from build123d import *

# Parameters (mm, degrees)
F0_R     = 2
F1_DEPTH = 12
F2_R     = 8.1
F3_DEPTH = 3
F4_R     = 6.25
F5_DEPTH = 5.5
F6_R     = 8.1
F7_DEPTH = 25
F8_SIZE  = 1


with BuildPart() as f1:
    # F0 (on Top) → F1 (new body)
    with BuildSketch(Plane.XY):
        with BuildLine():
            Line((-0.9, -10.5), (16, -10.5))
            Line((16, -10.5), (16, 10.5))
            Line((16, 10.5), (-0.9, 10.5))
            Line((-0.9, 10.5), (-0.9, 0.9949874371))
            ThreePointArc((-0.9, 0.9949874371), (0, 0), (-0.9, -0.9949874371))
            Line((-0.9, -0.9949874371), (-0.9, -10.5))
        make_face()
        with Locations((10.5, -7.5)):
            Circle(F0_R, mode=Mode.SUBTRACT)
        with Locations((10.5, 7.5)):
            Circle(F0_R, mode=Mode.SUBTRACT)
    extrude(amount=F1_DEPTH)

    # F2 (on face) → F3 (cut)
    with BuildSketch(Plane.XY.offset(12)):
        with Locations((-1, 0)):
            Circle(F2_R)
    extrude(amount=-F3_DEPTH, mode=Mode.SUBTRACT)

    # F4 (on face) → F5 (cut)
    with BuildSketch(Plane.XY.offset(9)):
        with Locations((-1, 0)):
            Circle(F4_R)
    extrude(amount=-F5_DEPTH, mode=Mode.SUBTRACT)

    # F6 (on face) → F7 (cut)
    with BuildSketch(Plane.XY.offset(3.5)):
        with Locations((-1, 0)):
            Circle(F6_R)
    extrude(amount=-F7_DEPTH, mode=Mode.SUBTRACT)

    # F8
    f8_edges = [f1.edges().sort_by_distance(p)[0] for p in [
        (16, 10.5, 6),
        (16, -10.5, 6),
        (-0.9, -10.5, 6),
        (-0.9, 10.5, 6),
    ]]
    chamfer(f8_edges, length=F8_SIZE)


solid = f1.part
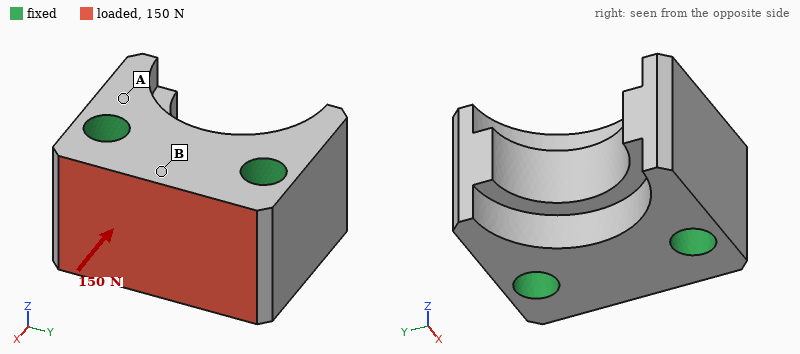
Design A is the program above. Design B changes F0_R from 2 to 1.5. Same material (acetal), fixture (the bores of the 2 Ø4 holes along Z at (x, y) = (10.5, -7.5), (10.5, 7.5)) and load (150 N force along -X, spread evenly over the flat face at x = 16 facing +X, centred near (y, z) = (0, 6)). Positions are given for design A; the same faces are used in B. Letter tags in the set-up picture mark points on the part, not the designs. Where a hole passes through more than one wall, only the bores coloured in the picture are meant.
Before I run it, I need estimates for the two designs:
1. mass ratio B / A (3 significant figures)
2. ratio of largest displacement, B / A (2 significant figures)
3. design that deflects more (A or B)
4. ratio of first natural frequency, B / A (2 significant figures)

1.04
1.2
B
0.92
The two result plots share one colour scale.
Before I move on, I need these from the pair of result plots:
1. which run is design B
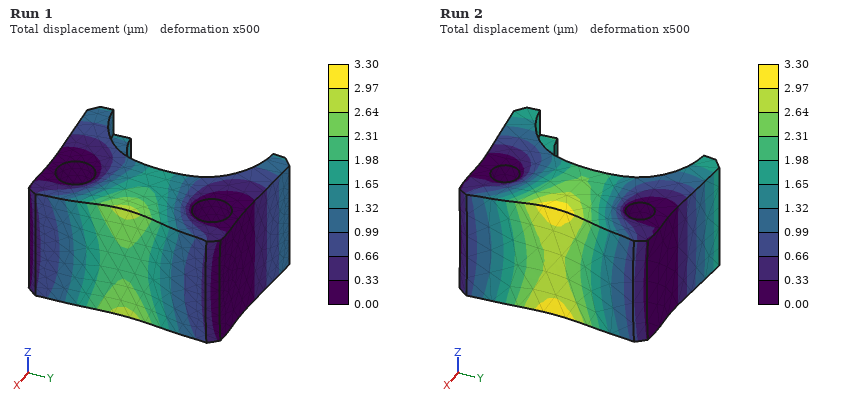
Run 2
